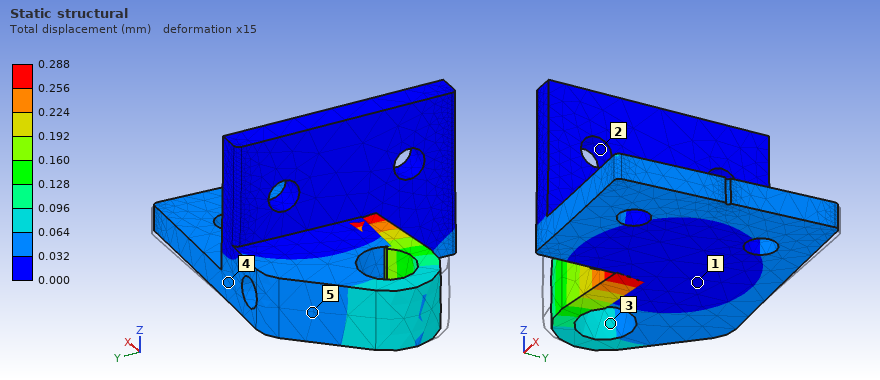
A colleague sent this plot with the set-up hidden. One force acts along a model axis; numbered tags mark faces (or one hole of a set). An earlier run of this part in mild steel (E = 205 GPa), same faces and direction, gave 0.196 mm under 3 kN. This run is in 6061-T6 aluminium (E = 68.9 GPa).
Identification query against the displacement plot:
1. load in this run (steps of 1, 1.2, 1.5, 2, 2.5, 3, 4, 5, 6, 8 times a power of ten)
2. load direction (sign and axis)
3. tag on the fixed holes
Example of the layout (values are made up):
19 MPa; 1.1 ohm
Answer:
1.5 kN; +Y; 2
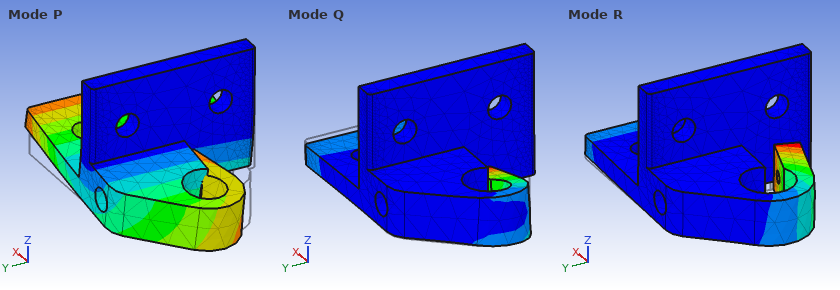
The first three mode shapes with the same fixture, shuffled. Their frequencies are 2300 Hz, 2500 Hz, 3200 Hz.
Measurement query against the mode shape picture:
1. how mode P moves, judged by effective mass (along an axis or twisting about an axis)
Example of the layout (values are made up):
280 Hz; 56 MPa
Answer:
along X
